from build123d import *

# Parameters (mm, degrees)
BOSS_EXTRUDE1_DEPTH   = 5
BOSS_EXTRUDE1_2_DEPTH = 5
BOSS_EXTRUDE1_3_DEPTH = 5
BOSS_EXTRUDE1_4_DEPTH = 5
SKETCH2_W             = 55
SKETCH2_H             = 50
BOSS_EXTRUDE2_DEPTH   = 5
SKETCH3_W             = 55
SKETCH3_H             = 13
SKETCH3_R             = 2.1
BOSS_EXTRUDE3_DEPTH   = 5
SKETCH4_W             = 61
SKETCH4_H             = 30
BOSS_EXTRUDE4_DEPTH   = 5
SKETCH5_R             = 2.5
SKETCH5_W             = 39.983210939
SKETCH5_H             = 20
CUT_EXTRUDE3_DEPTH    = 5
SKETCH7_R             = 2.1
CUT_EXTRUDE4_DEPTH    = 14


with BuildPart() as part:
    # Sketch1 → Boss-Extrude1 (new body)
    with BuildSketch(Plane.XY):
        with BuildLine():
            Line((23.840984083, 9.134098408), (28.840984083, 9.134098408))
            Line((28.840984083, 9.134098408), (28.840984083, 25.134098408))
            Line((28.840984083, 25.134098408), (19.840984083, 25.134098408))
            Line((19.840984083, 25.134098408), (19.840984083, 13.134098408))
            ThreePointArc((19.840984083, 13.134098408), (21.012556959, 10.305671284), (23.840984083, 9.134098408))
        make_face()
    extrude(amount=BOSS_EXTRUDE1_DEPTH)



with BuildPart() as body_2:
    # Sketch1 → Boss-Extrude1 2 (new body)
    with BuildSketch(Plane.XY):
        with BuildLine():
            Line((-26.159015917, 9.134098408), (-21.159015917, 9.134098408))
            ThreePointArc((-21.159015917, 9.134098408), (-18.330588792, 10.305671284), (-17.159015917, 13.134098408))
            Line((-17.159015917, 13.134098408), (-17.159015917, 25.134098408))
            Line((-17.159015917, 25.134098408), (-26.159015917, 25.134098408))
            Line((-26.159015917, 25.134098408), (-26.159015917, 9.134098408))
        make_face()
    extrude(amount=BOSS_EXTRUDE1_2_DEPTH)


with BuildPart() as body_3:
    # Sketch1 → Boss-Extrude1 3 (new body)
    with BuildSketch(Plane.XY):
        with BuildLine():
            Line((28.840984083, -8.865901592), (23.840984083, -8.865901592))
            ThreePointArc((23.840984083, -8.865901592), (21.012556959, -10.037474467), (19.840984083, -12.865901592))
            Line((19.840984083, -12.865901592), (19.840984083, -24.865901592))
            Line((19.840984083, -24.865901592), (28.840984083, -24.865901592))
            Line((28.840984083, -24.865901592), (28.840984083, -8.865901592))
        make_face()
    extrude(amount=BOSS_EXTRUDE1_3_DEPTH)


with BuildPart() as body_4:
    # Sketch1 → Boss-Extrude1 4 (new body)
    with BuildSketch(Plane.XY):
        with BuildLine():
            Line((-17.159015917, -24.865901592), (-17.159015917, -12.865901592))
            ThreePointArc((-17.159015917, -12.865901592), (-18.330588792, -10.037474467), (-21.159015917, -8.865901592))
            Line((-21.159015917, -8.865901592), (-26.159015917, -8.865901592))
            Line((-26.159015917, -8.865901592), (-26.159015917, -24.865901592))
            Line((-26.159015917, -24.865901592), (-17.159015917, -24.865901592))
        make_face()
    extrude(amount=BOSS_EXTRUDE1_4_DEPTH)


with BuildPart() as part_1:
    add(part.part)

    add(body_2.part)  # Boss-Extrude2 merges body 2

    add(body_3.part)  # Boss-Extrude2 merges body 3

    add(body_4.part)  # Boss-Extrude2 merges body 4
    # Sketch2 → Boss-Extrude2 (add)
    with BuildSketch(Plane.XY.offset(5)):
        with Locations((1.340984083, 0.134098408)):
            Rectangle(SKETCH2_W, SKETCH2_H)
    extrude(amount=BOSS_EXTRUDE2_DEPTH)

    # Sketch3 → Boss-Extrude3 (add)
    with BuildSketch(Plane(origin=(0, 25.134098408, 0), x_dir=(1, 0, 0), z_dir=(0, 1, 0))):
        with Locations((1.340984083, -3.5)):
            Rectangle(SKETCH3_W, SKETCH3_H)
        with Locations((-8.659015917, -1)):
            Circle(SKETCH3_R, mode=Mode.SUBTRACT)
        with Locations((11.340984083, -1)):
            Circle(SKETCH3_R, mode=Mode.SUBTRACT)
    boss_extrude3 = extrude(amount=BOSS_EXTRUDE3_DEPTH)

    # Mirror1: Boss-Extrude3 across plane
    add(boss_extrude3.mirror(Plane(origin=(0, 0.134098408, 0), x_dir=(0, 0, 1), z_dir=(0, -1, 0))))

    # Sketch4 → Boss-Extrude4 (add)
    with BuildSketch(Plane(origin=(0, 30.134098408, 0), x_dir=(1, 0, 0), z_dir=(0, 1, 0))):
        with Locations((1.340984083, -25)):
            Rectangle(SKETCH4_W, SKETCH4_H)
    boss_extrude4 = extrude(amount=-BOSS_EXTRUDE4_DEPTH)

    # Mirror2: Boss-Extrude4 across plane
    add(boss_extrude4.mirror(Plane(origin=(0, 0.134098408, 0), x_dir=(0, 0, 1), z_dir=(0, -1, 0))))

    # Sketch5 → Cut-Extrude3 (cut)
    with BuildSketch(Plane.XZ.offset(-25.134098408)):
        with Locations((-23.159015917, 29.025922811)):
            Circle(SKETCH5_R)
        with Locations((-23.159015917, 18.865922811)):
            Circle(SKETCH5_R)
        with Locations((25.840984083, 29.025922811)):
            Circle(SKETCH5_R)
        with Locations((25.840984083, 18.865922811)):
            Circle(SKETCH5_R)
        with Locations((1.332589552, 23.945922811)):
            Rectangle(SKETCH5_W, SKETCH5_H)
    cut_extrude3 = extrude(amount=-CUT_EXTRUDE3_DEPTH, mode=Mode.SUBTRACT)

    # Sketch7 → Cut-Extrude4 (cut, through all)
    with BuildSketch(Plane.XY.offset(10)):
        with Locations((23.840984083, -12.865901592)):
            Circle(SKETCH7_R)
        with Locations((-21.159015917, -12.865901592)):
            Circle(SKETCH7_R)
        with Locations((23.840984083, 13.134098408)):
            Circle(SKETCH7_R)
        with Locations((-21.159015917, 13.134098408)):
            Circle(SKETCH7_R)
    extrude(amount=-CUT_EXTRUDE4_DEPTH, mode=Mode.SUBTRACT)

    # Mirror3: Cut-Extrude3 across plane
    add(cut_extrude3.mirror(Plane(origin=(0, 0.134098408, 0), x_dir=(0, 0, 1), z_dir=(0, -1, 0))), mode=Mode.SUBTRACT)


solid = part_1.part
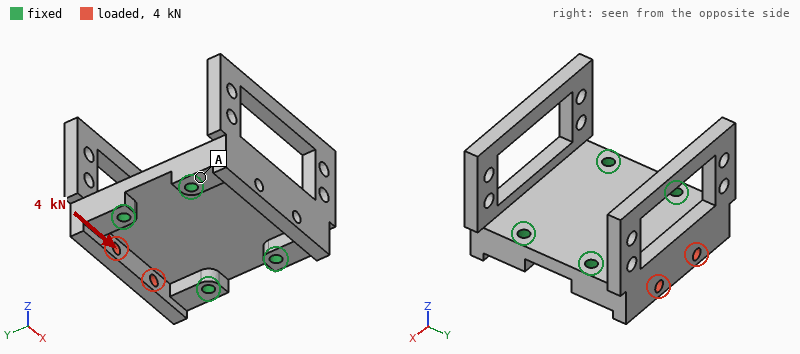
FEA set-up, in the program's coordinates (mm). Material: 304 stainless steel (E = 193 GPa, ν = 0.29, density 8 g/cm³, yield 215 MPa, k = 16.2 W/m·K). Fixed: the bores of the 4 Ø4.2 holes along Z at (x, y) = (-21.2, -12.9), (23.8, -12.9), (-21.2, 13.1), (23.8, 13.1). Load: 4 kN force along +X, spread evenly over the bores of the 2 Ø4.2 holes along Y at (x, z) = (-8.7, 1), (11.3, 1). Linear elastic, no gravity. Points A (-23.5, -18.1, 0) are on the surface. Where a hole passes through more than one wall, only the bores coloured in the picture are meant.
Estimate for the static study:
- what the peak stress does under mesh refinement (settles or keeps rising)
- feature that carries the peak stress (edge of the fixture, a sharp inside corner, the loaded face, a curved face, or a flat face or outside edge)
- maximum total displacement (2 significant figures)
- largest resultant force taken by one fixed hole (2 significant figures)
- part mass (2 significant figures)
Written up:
keeps rising
edge of the fixture
10 µm
2.2 kN
260 g
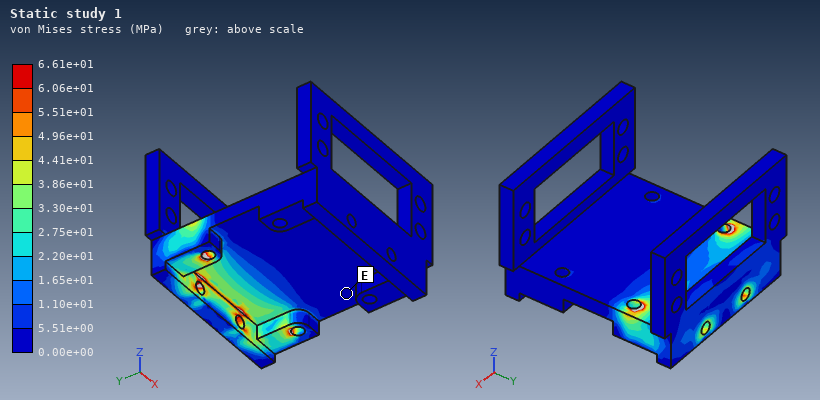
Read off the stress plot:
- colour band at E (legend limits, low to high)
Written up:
0.00e+00 to 5.51e+00 MPa
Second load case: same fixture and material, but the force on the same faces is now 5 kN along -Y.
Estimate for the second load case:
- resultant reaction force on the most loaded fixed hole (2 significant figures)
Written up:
2.1 kN
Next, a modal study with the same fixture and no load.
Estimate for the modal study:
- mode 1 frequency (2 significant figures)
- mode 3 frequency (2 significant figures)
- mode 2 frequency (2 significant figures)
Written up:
2100 Hz
3800 Hz
2100 Hz
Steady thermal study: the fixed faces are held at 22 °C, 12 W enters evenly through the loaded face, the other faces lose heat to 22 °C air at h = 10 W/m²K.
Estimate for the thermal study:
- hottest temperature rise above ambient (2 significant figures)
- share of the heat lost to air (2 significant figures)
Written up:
69 K
14 %
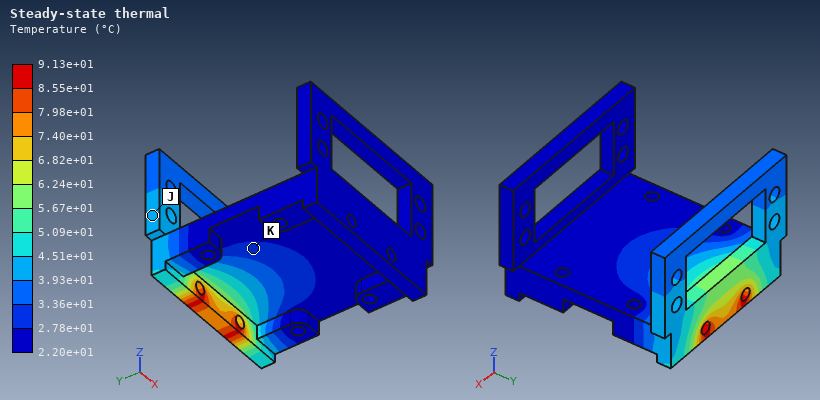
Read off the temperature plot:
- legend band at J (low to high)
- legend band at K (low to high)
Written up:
3.93e+01 to 4.51e+01 °C
2.78e+01 to 3.36e+01 °C
